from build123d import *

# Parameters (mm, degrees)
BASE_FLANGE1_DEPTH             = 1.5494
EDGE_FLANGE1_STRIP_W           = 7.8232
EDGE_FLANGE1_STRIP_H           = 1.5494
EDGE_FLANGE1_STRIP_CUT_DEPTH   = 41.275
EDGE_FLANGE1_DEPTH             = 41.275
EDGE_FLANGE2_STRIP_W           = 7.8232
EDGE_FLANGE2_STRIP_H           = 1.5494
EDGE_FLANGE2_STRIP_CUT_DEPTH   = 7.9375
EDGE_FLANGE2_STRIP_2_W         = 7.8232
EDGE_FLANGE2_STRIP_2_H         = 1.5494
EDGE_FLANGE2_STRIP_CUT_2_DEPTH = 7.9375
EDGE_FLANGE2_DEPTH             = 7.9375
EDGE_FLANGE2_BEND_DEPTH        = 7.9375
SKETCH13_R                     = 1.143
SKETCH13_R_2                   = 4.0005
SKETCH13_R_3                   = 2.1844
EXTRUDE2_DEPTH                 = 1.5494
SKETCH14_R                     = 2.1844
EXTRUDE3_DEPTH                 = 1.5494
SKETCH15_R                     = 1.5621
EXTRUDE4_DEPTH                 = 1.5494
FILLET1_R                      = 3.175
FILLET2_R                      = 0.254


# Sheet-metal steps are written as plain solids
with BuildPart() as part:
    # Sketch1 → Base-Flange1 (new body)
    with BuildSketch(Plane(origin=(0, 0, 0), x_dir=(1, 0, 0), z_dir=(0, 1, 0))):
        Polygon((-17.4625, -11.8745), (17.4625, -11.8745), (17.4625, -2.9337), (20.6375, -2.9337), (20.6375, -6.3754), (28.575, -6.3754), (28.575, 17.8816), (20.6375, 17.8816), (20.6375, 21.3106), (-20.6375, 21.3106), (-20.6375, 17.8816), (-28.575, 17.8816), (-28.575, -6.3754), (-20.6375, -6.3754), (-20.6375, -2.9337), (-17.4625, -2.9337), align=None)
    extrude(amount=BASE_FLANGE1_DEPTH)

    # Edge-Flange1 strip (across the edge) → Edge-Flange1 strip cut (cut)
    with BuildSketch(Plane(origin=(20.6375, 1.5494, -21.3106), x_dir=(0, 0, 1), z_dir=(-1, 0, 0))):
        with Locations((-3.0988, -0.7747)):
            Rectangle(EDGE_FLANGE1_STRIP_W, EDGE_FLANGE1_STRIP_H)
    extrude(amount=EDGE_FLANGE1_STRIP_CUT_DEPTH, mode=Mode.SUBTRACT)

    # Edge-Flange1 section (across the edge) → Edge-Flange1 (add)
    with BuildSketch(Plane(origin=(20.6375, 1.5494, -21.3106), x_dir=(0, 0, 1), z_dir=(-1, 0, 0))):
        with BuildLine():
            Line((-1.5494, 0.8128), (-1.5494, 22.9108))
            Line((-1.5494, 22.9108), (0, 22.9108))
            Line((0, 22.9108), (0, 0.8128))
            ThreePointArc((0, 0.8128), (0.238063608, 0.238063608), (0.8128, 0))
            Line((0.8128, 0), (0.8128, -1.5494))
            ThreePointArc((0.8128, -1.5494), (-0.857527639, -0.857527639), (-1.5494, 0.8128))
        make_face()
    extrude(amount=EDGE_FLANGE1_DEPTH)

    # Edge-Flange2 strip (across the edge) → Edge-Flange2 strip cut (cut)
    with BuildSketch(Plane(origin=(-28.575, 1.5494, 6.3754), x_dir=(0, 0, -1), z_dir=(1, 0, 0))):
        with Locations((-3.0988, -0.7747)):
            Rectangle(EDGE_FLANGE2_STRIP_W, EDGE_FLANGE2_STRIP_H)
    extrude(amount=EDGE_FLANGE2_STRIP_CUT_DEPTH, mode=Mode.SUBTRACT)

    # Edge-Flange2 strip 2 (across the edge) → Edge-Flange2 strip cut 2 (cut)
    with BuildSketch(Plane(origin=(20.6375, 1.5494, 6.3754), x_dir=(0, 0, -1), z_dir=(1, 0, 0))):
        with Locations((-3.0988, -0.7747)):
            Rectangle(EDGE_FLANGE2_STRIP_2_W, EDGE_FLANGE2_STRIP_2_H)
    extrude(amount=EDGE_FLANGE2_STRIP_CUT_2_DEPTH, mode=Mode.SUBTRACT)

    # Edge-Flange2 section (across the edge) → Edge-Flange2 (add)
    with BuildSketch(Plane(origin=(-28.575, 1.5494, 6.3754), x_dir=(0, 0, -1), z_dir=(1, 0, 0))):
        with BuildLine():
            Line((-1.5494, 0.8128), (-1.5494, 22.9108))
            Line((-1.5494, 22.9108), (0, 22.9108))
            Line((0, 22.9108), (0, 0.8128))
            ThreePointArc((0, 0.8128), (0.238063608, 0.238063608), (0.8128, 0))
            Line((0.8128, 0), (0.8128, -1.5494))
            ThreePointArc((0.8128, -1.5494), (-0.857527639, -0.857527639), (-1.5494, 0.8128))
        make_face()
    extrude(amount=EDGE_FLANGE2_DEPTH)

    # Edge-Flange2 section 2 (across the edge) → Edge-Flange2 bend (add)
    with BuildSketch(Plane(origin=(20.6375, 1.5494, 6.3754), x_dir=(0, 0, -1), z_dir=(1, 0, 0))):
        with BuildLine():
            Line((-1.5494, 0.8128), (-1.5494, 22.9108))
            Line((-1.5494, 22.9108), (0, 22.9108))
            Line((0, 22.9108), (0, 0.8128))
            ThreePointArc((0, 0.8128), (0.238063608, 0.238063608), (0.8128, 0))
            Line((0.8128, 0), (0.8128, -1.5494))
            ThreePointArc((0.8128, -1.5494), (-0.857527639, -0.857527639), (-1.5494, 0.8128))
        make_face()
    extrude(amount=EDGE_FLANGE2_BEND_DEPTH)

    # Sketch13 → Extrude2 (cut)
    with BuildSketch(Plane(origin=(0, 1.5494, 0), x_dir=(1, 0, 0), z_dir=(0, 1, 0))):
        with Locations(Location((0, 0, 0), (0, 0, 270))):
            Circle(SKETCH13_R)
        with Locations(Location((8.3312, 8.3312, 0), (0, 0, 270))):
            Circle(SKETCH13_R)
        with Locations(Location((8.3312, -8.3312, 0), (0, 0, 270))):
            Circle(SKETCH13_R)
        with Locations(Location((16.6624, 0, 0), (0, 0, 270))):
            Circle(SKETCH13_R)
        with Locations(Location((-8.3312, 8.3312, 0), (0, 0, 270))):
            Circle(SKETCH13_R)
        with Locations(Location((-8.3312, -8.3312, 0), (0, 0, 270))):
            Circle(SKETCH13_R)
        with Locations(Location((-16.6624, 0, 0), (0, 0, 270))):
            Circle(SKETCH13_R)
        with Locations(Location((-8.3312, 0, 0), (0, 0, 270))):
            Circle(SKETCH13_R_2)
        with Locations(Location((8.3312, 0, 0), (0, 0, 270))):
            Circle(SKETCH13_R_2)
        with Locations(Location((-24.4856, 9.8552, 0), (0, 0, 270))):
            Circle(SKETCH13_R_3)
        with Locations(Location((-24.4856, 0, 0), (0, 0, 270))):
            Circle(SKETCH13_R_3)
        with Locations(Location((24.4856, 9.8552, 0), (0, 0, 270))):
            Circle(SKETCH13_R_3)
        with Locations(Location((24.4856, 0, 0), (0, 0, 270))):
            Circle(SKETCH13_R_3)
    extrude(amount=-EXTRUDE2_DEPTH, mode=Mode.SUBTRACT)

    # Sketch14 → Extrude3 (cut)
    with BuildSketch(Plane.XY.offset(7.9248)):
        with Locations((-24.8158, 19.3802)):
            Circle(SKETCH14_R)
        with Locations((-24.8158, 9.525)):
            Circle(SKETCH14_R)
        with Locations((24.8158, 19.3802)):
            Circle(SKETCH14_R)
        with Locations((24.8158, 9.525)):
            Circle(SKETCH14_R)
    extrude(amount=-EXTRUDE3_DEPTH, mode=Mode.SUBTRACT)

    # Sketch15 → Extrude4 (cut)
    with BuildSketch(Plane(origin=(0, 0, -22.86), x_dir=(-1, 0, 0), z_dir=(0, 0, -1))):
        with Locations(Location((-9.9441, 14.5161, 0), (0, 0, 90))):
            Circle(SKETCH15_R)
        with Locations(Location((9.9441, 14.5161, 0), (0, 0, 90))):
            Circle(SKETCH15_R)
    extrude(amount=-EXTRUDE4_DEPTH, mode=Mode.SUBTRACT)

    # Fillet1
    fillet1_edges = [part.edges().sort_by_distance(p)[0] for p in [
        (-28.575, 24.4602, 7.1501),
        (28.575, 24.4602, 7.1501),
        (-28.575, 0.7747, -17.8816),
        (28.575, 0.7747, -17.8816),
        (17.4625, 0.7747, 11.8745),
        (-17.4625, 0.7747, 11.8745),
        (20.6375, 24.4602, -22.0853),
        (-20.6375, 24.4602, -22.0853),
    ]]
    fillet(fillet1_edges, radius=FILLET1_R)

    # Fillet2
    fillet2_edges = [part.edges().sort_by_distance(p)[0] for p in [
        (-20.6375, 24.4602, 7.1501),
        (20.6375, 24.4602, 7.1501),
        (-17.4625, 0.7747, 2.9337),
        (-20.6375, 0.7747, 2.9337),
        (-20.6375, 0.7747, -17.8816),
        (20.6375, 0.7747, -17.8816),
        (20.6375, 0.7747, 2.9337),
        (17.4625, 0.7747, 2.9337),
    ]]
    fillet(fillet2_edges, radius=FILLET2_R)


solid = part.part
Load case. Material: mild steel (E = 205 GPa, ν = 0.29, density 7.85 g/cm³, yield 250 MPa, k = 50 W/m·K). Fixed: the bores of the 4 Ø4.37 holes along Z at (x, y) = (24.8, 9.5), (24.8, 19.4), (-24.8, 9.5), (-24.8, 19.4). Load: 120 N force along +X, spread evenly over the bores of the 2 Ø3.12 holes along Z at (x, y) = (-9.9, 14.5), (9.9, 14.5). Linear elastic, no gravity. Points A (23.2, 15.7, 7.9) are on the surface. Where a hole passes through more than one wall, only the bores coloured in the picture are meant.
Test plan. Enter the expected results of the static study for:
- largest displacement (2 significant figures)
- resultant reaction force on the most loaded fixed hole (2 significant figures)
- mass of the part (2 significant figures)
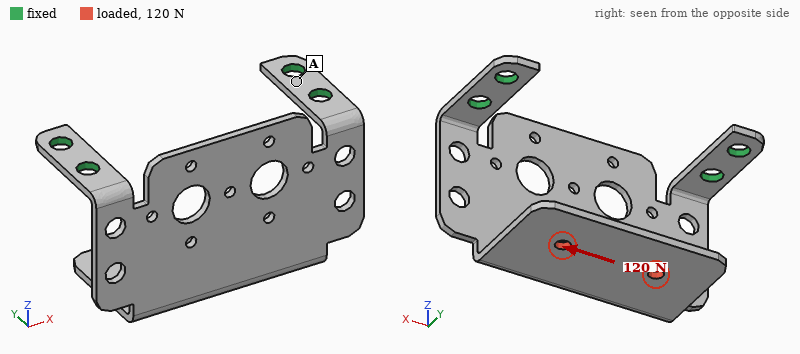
0.26 mm
97 N
34 g
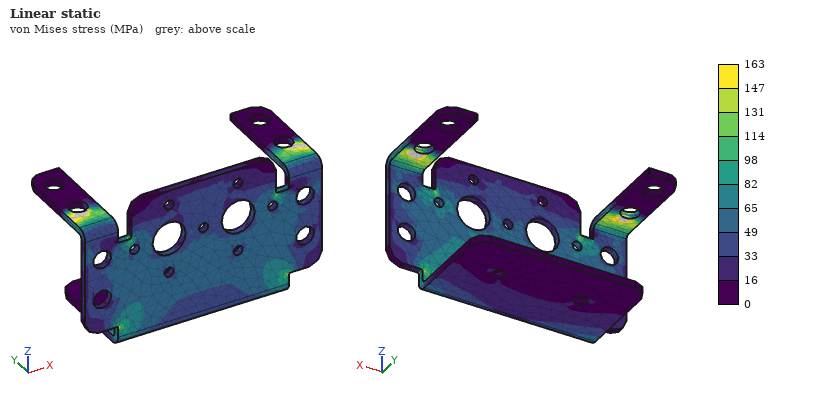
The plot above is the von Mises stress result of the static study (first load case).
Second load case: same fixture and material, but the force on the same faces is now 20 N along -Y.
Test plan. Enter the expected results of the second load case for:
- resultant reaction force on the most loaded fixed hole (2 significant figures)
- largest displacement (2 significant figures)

9.8 N
0.35 mm
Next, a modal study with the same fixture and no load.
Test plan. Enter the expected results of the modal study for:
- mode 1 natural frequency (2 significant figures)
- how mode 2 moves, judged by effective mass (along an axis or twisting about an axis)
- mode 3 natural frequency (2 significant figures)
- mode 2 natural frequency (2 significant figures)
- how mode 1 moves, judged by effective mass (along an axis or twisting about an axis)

320 Hz
along X
1300 Hz
1000 Hz
along Y
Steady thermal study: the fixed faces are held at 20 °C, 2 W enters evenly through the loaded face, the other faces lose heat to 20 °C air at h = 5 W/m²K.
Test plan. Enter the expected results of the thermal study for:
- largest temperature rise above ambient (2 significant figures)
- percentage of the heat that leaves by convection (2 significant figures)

39 K
37 %
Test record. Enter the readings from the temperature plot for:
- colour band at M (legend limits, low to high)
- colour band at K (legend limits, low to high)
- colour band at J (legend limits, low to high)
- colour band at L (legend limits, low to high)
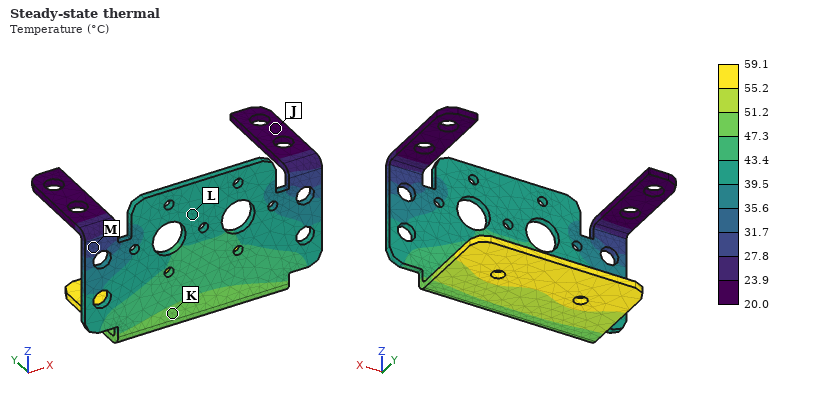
27.8 to 31.7 °C
47.3 to 51.2 °C
20.0 to 23.9 °C
39.5 to 43.4 °C
